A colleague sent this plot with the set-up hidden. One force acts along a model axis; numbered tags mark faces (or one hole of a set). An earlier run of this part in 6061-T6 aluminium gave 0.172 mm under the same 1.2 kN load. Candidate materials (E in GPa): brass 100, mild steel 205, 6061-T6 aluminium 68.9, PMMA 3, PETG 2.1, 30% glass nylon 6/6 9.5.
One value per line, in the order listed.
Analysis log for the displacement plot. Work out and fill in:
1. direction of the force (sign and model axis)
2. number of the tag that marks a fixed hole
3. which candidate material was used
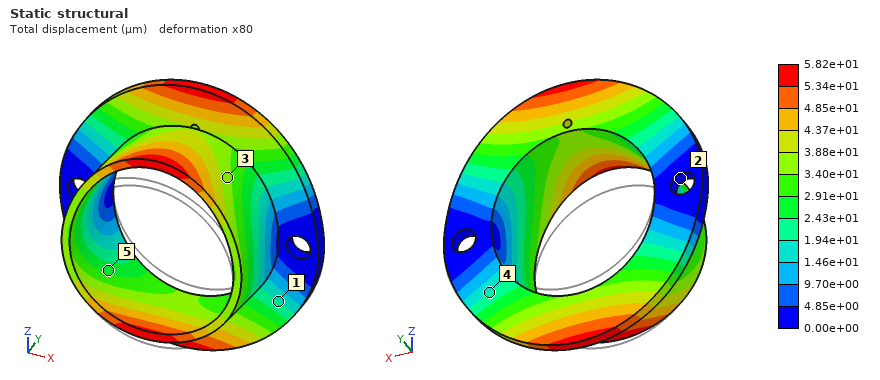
+Z
2
mild steel
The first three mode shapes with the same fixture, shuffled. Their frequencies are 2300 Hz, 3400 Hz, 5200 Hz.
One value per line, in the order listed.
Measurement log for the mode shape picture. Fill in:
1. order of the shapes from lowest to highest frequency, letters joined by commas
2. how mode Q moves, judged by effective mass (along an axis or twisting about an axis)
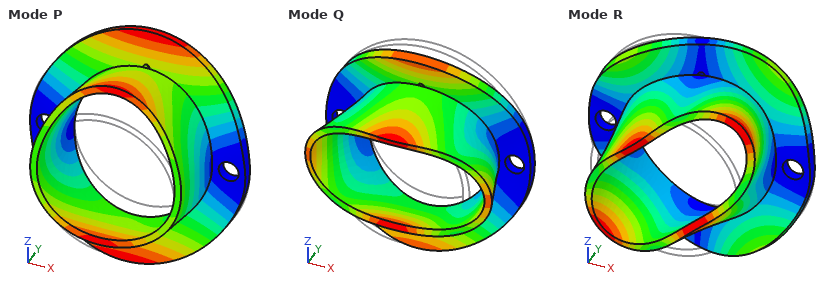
P, Q, R
along Y
